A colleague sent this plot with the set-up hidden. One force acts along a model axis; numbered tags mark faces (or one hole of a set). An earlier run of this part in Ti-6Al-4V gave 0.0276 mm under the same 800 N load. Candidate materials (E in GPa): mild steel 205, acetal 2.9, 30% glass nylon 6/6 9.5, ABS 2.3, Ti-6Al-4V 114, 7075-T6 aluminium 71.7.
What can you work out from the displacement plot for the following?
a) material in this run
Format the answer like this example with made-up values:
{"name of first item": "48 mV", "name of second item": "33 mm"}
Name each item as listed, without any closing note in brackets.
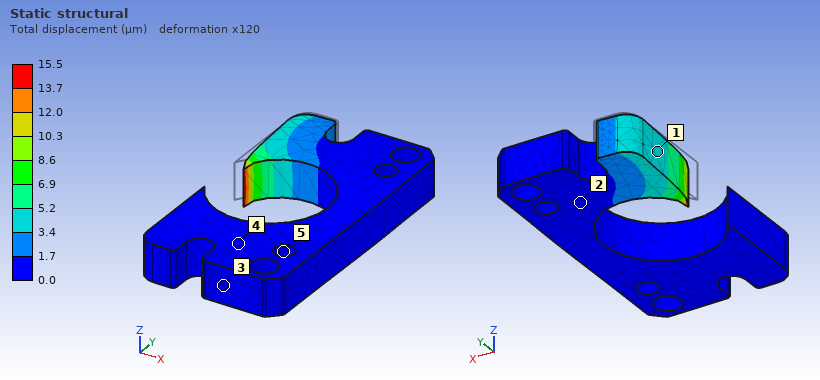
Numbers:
{"material in this run": "mild steel"}
